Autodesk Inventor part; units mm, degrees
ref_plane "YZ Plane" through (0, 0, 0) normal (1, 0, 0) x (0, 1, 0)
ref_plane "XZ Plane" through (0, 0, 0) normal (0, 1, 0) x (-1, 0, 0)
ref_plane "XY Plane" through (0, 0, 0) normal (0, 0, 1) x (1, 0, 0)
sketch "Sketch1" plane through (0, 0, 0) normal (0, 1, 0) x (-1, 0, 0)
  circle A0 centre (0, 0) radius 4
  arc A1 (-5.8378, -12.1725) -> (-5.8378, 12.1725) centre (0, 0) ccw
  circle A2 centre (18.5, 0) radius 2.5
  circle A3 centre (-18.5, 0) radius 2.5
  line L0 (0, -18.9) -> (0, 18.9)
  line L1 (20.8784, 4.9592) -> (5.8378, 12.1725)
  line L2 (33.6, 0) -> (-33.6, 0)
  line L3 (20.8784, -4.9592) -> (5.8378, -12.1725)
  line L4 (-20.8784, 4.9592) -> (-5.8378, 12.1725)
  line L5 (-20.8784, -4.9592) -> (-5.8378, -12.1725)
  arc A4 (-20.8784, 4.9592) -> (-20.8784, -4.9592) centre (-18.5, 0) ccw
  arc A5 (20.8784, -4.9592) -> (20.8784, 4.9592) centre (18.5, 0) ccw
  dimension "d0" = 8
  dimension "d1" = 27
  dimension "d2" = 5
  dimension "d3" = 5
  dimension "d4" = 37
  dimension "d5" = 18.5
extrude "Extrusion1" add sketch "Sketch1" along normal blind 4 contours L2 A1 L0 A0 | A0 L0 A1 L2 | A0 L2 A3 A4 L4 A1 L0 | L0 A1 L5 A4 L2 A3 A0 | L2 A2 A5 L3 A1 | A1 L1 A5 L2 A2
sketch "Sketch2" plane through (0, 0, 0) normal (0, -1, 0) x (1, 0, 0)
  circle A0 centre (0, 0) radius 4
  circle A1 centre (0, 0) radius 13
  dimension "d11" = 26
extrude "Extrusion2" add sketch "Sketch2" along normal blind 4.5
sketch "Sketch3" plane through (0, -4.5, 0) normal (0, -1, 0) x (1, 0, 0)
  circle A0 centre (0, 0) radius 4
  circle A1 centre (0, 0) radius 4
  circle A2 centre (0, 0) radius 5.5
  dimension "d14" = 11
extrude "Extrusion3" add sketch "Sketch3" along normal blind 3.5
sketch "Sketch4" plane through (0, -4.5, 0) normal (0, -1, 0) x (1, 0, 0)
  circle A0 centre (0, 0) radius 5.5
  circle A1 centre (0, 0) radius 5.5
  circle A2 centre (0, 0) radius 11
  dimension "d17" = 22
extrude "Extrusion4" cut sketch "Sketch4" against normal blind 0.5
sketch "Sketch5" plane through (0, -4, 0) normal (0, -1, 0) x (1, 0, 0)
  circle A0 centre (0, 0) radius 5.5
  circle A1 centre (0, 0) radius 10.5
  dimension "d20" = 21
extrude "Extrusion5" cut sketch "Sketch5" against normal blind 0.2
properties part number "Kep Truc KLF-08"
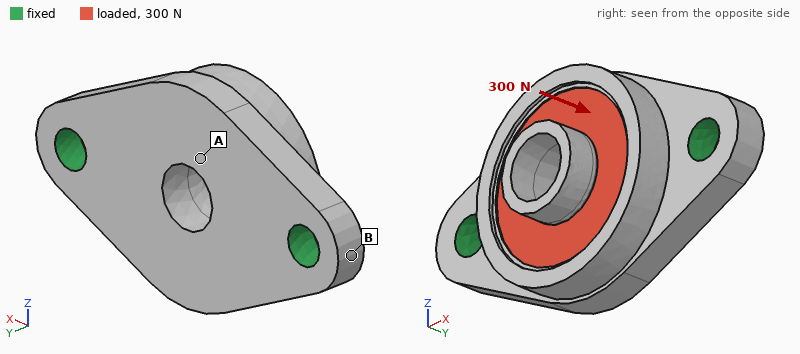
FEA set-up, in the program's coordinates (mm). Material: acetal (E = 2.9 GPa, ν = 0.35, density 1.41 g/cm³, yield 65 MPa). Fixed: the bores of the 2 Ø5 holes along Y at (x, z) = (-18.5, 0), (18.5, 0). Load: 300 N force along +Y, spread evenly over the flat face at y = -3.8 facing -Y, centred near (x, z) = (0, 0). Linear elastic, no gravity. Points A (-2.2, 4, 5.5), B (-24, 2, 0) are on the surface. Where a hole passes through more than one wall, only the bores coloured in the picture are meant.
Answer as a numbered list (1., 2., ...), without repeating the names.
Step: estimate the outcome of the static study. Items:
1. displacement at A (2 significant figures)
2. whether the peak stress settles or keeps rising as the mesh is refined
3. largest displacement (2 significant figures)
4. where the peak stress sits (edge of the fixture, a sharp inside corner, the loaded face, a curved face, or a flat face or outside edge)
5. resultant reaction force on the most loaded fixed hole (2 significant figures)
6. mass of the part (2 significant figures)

1. 74 µm
2. keeps rising
3. 89 µm
4. edge of the fixture
5. 180 N
6. 7.4 g
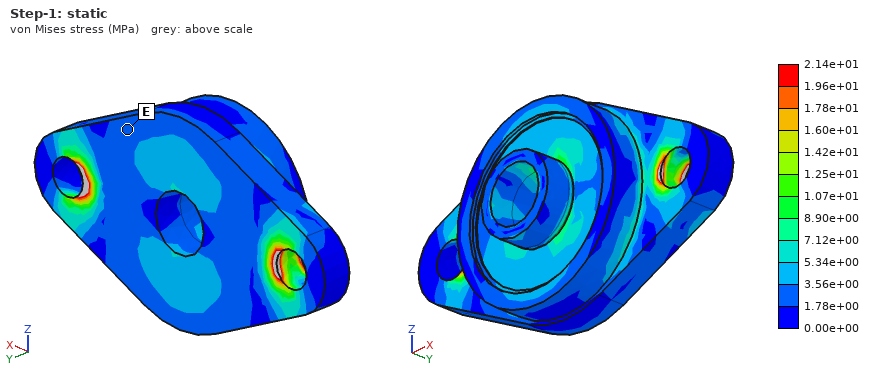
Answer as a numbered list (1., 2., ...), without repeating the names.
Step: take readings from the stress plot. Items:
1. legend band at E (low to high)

1. 1.78e+00 to 3.56e+00 MPa
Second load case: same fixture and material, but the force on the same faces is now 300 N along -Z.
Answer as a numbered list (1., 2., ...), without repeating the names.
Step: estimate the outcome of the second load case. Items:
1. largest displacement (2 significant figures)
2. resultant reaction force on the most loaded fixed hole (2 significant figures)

1. 0.22 mm
2. 150 N
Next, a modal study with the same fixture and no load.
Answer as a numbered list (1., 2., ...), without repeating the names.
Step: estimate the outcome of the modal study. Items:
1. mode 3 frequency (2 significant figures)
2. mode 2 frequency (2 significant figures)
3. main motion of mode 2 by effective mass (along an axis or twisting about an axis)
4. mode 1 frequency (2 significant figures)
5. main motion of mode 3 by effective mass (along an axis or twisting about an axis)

1. 7500 Hz
2. 4200 Hz
3. along Y
4. 2900 Hz
5. along Z
